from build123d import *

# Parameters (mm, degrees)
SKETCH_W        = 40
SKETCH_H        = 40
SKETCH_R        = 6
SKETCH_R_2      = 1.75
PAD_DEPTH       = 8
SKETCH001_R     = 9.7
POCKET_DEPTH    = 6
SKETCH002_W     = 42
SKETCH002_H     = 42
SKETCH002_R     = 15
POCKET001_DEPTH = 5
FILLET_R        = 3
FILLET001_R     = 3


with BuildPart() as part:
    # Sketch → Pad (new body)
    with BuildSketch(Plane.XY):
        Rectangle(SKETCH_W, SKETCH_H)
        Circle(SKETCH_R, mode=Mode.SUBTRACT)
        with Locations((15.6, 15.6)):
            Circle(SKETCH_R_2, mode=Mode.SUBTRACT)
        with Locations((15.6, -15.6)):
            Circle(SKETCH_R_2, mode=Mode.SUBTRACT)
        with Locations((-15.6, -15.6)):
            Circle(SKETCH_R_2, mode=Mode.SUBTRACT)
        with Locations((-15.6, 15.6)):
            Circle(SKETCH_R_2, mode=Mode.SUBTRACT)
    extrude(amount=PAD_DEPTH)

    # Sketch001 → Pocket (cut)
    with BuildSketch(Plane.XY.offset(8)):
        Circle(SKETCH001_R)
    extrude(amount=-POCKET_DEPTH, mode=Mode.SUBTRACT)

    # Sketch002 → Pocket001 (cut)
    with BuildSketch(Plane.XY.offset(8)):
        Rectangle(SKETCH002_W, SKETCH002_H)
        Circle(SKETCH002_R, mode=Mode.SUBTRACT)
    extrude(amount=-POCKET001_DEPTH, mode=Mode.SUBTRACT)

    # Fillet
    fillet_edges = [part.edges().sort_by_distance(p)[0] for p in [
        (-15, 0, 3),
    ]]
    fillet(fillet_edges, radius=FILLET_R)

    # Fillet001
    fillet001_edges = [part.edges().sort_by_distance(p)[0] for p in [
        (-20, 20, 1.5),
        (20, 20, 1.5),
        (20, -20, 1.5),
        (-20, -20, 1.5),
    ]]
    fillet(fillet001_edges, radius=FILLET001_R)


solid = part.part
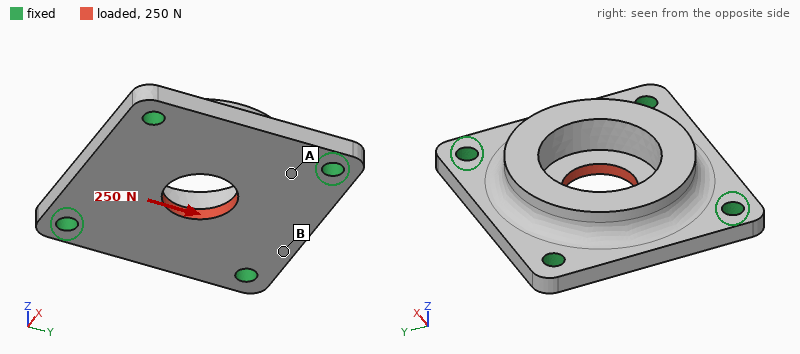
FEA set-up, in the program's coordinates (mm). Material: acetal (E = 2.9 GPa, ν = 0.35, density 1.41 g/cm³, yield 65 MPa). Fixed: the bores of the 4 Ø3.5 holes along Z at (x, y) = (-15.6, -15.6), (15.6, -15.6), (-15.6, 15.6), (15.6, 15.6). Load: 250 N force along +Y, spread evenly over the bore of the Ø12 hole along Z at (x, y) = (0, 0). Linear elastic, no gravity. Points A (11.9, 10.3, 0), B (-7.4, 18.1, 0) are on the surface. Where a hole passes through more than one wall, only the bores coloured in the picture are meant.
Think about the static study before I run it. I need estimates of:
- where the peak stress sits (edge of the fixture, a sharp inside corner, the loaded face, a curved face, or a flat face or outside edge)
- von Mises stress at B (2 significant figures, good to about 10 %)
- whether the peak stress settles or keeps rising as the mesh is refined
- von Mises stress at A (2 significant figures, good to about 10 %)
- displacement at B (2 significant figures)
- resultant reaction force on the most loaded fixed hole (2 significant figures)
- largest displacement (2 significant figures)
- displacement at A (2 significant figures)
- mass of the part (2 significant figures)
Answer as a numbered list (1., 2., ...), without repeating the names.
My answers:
1. edge of the fixture
2. 0.97 MPa
3. keeps rising
4. 2.4 MPa
5. 11 µm
6. 68 N
7. 22 µm
8. 5.6 µm
9. 9.0 g
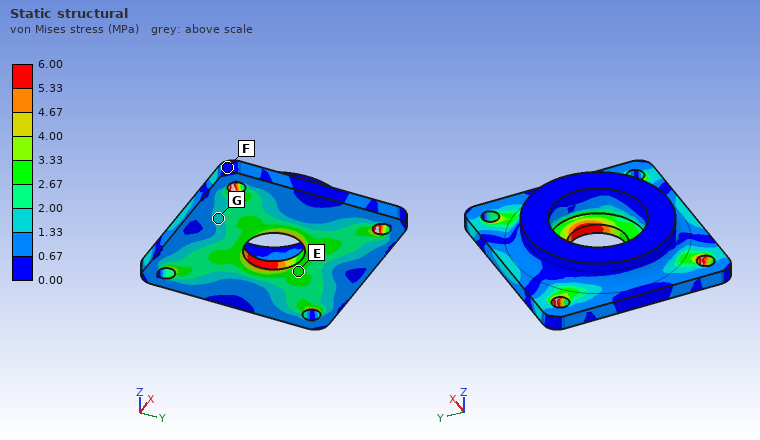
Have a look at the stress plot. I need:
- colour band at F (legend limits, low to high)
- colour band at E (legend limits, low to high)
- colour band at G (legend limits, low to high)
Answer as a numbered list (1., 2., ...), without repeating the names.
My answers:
1. 0.00 to 0.67 MPa
2. 2.67 to 3.33 MPa
3. 1.33 to 2.00 MPa
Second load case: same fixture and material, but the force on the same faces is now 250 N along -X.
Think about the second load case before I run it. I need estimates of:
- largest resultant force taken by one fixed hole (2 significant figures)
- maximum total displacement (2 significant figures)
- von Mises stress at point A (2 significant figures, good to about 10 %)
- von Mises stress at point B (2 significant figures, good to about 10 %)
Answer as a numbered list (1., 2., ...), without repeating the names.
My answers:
1. 68 N
2. 22 µm
3. 2.6 MPa
4. 0.91 MPa
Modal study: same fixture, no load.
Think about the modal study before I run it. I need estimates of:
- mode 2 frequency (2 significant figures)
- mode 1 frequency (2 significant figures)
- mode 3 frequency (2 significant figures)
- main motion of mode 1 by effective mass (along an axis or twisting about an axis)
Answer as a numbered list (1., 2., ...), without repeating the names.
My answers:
1. 5800 Hz
2. 4400 Hz
3. 5800 Hz
4. along Z
